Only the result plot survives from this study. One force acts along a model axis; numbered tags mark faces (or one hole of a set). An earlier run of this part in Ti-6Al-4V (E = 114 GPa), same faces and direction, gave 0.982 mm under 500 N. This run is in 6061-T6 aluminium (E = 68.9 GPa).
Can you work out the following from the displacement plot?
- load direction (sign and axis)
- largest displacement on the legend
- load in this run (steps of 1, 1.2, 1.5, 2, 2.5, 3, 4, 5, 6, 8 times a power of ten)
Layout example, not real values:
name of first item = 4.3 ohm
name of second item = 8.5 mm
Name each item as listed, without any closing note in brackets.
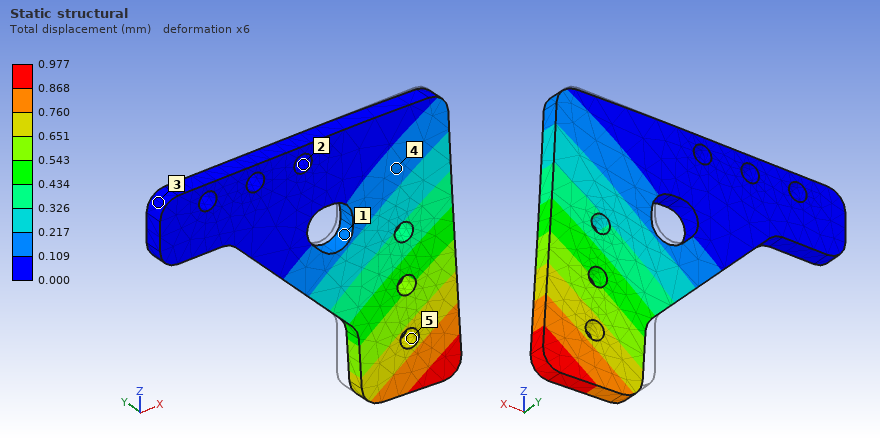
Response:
load direction = -Y
largest displacement on the legend = 0.977 mm
load in this run = 300 N
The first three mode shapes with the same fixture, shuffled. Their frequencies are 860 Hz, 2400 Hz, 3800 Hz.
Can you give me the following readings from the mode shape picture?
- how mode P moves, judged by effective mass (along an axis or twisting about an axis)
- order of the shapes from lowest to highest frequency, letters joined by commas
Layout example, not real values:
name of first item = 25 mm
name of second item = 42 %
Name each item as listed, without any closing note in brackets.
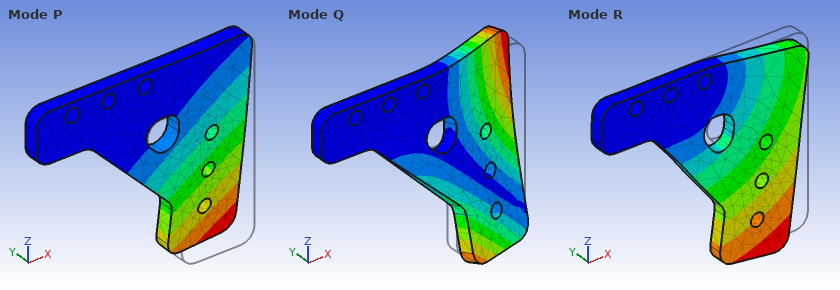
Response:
how mode P moves, judged by effective mass = along Y
order of the shapes from lowest to highest frequency, letters joined by commas = P, Q, R
